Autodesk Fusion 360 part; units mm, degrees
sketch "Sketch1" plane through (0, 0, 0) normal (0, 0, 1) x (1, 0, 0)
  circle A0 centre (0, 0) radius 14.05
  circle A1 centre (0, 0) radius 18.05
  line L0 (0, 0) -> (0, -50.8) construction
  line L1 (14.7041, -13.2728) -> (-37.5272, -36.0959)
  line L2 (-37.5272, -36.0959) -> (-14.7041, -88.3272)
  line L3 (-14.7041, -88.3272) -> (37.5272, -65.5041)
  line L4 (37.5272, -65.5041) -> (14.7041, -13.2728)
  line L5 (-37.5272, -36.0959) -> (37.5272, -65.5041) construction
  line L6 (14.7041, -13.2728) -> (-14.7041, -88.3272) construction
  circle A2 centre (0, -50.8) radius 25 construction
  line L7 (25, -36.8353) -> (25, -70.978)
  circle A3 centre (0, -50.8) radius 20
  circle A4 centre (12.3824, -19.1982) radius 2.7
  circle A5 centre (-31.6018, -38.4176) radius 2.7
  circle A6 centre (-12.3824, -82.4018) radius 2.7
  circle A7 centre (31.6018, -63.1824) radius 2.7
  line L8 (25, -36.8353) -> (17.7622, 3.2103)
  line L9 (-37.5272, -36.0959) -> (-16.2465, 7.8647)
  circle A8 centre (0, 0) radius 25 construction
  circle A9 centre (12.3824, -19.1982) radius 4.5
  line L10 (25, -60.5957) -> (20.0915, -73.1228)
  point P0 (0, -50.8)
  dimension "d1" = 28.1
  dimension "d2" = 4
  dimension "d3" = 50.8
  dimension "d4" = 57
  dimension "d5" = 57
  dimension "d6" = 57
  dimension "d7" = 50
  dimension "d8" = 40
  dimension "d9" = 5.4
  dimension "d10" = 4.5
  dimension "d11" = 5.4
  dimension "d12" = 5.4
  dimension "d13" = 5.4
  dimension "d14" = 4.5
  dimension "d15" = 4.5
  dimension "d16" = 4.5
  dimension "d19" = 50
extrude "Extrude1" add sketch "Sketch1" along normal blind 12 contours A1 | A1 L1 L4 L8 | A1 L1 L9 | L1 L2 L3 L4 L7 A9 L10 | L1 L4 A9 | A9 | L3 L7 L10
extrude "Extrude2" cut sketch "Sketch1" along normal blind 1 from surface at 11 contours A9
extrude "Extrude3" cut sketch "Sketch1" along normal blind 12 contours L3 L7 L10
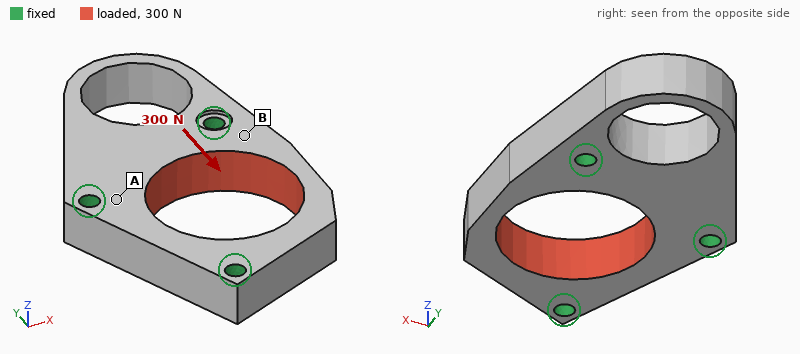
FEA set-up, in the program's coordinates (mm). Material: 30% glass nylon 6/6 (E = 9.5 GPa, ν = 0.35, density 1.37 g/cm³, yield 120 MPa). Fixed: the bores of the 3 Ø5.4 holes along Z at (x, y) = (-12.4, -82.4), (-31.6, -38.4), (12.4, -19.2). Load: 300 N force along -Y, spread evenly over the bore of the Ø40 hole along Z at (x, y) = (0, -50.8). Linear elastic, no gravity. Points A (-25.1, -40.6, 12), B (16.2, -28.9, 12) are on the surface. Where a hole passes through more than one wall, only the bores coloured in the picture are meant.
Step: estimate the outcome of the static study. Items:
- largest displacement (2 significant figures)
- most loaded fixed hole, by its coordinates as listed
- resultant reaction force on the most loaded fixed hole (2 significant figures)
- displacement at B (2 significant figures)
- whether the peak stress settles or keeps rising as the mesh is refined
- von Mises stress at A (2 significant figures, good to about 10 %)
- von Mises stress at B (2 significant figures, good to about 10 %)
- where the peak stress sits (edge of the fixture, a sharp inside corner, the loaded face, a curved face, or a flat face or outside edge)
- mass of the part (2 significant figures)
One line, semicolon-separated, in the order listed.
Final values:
5.4 µm; (12.4, -19.2); 140 N; 1.00 µm; keeps rising; 0.23 MPa; 0.67 MPa; edge of the fixture; 44 g
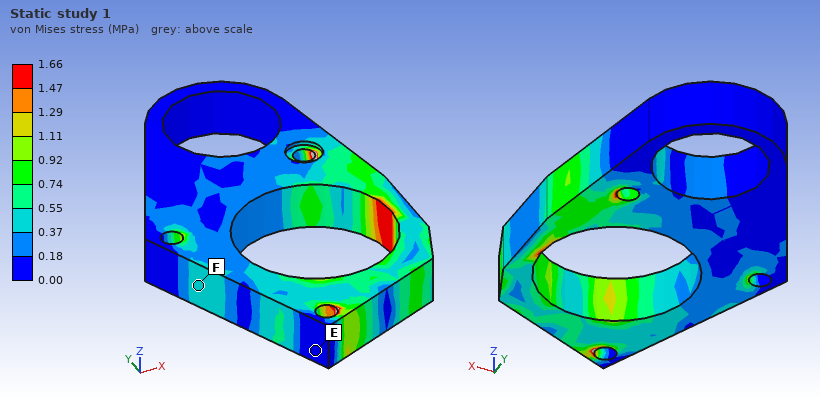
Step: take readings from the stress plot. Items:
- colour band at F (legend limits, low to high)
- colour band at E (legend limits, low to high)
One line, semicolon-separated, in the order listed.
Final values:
0.37 to 0.55 MPa; 0.00 to 0.18 MPa
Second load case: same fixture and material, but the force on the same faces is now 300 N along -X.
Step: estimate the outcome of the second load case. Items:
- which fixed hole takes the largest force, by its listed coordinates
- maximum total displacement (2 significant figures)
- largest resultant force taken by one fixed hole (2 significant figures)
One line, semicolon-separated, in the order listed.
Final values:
(-12.4, -82.4); 6.2 µm; 130 N
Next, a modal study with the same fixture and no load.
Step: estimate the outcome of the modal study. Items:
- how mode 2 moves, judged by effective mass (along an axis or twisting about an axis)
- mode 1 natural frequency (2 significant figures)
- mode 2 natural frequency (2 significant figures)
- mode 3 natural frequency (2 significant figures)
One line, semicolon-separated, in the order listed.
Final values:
along Z; 3100 Hz; 4300 Hz; 5000 Hz
